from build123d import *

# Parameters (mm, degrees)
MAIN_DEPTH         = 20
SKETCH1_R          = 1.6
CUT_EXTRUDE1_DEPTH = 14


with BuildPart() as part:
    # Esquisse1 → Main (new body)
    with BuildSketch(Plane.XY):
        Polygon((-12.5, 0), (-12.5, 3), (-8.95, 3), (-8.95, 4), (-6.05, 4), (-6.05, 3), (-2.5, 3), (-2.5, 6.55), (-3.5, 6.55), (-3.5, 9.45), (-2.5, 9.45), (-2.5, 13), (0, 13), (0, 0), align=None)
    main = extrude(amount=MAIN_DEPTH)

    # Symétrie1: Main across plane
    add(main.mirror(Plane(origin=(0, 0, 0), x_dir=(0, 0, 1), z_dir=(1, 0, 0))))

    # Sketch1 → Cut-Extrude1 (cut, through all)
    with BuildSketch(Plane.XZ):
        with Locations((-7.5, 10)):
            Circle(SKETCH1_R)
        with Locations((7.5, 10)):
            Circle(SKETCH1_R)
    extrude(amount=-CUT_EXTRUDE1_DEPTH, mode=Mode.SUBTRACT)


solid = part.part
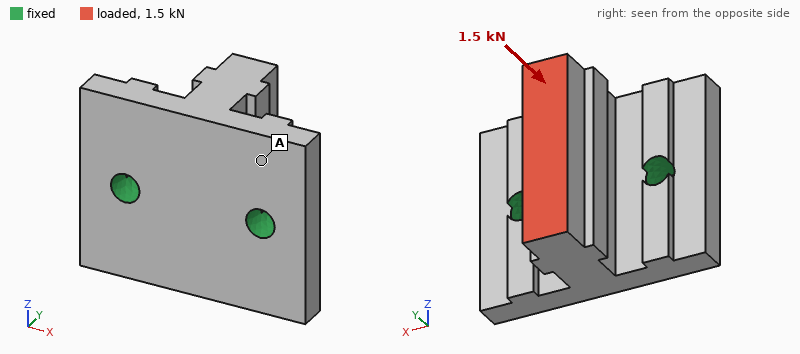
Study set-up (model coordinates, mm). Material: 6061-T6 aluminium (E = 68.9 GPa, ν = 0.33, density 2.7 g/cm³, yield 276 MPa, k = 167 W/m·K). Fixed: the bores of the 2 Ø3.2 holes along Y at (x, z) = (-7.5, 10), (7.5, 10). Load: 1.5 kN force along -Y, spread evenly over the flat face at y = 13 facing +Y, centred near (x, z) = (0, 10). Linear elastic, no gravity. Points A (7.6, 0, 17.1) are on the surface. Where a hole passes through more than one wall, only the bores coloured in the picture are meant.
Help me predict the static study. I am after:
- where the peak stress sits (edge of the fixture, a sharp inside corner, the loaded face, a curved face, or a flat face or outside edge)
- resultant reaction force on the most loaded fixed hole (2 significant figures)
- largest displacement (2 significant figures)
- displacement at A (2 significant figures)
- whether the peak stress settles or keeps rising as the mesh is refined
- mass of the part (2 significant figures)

edge of the fixture
760 N
13 µm
5.0 µm
keeps rising
7.2 g
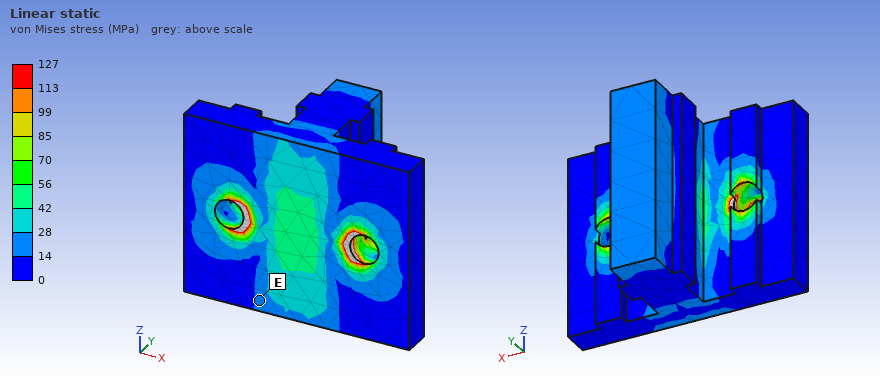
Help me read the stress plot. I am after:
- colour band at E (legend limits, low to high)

14 to 28 MPa
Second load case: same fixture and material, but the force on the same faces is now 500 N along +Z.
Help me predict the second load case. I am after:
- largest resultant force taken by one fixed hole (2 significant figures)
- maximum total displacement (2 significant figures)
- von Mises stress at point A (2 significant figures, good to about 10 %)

250 N
38 µm
19 MPa
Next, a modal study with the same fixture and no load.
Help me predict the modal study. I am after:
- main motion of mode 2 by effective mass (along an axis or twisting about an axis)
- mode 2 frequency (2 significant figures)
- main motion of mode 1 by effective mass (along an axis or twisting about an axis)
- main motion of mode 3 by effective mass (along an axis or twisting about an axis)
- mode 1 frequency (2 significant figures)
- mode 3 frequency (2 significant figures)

along X
20 kHz
along Z
along Y
14 kHz
27 kHz
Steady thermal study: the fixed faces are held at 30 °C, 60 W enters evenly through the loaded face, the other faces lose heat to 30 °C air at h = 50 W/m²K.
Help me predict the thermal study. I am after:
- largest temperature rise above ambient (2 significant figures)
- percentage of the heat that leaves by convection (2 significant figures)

58 K
3.1 %
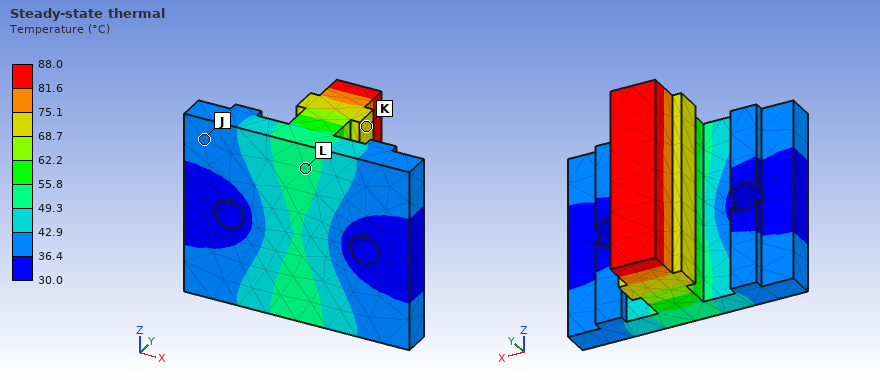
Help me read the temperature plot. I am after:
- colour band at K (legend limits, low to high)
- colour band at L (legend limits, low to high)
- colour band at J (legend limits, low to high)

68.7 to 75.1 °C
49.3 to 55.8 °C
36.4 to 42.9 °C
